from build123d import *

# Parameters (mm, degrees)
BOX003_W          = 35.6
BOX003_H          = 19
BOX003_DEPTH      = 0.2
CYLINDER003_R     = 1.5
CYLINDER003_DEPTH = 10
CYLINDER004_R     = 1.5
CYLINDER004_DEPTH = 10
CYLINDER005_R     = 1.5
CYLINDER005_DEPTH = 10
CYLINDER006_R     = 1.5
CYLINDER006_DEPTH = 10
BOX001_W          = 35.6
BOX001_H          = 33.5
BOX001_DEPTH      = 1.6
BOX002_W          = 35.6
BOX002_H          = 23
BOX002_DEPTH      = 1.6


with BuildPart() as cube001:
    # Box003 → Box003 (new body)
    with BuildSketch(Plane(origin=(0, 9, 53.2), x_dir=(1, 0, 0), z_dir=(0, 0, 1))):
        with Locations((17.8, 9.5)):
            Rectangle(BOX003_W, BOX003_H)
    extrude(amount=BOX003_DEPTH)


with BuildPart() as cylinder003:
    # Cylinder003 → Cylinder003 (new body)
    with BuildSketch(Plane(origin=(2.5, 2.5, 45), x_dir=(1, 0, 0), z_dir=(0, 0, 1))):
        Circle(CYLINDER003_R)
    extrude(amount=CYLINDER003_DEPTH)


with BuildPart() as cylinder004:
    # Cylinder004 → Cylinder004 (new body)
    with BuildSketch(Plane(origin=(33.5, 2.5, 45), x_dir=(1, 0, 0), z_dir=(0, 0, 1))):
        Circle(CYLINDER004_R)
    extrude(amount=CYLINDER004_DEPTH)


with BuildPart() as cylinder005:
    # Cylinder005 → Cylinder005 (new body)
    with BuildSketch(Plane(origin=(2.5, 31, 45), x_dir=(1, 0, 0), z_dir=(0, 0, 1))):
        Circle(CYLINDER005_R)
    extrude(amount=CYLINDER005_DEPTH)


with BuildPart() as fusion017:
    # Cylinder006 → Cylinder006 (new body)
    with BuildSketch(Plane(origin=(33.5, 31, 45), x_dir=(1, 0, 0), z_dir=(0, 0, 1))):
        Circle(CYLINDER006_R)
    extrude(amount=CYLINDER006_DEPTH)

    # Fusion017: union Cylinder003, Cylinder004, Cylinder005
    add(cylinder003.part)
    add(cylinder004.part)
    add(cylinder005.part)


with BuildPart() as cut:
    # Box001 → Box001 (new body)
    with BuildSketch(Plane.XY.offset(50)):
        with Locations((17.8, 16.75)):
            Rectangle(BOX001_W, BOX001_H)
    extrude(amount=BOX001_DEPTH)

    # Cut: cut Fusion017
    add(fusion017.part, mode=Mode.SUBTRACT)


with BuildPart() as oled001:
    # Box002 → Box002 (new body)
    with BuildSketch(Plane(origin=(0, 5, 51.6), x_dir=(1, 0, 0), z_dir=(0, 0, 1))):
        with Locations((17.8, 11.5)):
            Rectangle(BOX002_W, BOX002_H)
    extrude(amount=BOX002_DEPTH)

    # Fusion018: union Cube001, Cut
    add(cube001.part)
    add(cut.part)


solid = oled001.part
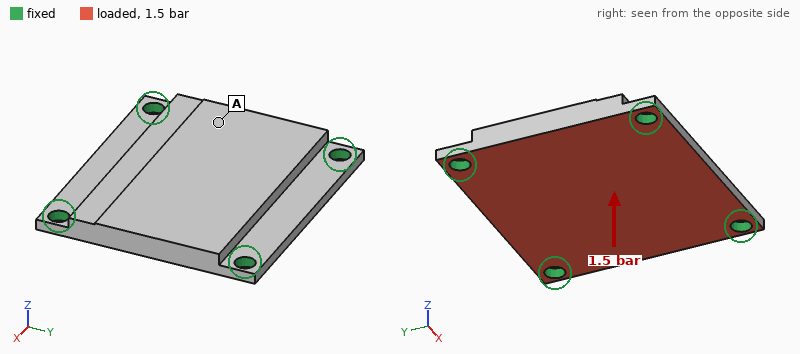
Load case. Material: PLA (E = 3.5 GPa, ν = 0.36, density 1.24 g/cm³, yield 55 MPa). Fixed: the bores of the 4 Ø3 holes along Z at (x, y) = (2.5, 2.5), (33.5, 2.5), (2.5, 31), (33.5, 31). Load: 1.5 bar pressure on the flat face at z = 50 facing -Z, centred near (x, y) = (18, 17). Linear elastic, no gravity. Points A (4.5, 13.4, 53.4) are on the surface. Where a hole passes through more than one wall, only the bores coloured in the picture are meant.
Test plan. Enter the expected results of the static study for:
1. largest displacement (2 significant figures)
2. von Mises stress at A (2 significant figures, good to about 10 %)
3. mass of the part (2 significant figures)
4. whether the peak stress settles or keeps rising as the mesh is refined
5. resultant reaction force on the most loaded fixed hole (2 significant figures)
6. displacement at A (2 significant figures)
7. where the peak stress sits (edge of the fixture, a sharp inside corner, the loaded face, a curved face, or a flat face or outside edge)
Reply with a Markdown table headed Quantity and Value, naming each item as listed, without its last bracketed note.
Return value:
| Quantity | Value |
|---|---|
| largest displacement | 0.15 mm |
| von Mises stress at A | 4.8 MPa |
| mass of the part | 4.1 g |
| whether the peak stress settles or keeps rising as the mesh is refined | keeps rising |
| resultant reaction force on the most loaded fixed hole | 65 N |
| displacement at A | 0.068 mm |
| where the peak stress sits | edge of the fixture |
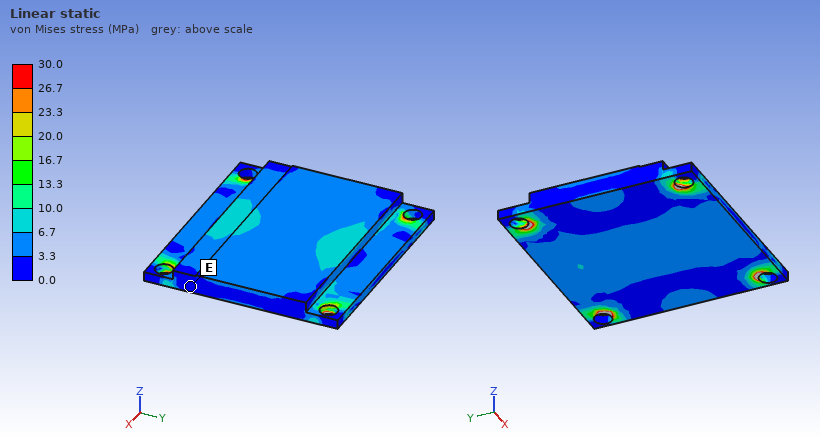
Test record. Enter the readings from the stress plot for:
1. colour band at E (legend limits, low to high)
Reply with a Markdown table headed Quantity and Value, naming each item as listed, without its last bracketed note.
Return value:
| Quantity | Value |
|---|---|
| colour band at E | 0.0 to 3.3 MPa |
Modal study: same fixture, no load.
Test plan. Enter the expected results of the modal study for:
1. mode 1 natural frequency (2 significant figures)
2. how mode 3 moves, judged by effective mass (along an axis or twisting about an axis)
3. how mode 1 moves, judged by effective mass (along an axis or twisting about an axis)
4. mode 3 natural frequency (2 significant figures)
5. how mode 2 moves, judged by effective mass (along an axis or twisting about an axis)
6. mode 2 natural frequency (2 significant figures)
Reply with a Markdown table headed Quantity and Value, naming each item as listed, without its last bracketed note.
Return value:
| Quantity | Value |
|---|---|
| mode 1 natural frequency | 3200 Hz |
| how mode 3 moves, judged by effective mass | twisting about Y |
| how mode 1 moves, judged by effective mass | along Z |
| mode 3 natural frequency | 5900 Hz |
| how mode 2 moves, judged by effective mass | twisting about X |
| mode 2 natural frequency | 5000 Hz |
